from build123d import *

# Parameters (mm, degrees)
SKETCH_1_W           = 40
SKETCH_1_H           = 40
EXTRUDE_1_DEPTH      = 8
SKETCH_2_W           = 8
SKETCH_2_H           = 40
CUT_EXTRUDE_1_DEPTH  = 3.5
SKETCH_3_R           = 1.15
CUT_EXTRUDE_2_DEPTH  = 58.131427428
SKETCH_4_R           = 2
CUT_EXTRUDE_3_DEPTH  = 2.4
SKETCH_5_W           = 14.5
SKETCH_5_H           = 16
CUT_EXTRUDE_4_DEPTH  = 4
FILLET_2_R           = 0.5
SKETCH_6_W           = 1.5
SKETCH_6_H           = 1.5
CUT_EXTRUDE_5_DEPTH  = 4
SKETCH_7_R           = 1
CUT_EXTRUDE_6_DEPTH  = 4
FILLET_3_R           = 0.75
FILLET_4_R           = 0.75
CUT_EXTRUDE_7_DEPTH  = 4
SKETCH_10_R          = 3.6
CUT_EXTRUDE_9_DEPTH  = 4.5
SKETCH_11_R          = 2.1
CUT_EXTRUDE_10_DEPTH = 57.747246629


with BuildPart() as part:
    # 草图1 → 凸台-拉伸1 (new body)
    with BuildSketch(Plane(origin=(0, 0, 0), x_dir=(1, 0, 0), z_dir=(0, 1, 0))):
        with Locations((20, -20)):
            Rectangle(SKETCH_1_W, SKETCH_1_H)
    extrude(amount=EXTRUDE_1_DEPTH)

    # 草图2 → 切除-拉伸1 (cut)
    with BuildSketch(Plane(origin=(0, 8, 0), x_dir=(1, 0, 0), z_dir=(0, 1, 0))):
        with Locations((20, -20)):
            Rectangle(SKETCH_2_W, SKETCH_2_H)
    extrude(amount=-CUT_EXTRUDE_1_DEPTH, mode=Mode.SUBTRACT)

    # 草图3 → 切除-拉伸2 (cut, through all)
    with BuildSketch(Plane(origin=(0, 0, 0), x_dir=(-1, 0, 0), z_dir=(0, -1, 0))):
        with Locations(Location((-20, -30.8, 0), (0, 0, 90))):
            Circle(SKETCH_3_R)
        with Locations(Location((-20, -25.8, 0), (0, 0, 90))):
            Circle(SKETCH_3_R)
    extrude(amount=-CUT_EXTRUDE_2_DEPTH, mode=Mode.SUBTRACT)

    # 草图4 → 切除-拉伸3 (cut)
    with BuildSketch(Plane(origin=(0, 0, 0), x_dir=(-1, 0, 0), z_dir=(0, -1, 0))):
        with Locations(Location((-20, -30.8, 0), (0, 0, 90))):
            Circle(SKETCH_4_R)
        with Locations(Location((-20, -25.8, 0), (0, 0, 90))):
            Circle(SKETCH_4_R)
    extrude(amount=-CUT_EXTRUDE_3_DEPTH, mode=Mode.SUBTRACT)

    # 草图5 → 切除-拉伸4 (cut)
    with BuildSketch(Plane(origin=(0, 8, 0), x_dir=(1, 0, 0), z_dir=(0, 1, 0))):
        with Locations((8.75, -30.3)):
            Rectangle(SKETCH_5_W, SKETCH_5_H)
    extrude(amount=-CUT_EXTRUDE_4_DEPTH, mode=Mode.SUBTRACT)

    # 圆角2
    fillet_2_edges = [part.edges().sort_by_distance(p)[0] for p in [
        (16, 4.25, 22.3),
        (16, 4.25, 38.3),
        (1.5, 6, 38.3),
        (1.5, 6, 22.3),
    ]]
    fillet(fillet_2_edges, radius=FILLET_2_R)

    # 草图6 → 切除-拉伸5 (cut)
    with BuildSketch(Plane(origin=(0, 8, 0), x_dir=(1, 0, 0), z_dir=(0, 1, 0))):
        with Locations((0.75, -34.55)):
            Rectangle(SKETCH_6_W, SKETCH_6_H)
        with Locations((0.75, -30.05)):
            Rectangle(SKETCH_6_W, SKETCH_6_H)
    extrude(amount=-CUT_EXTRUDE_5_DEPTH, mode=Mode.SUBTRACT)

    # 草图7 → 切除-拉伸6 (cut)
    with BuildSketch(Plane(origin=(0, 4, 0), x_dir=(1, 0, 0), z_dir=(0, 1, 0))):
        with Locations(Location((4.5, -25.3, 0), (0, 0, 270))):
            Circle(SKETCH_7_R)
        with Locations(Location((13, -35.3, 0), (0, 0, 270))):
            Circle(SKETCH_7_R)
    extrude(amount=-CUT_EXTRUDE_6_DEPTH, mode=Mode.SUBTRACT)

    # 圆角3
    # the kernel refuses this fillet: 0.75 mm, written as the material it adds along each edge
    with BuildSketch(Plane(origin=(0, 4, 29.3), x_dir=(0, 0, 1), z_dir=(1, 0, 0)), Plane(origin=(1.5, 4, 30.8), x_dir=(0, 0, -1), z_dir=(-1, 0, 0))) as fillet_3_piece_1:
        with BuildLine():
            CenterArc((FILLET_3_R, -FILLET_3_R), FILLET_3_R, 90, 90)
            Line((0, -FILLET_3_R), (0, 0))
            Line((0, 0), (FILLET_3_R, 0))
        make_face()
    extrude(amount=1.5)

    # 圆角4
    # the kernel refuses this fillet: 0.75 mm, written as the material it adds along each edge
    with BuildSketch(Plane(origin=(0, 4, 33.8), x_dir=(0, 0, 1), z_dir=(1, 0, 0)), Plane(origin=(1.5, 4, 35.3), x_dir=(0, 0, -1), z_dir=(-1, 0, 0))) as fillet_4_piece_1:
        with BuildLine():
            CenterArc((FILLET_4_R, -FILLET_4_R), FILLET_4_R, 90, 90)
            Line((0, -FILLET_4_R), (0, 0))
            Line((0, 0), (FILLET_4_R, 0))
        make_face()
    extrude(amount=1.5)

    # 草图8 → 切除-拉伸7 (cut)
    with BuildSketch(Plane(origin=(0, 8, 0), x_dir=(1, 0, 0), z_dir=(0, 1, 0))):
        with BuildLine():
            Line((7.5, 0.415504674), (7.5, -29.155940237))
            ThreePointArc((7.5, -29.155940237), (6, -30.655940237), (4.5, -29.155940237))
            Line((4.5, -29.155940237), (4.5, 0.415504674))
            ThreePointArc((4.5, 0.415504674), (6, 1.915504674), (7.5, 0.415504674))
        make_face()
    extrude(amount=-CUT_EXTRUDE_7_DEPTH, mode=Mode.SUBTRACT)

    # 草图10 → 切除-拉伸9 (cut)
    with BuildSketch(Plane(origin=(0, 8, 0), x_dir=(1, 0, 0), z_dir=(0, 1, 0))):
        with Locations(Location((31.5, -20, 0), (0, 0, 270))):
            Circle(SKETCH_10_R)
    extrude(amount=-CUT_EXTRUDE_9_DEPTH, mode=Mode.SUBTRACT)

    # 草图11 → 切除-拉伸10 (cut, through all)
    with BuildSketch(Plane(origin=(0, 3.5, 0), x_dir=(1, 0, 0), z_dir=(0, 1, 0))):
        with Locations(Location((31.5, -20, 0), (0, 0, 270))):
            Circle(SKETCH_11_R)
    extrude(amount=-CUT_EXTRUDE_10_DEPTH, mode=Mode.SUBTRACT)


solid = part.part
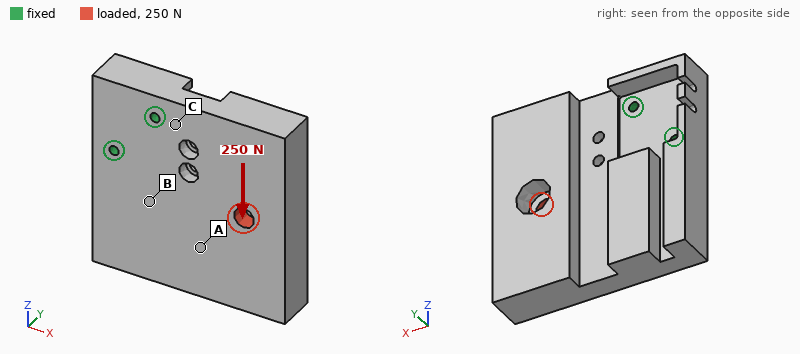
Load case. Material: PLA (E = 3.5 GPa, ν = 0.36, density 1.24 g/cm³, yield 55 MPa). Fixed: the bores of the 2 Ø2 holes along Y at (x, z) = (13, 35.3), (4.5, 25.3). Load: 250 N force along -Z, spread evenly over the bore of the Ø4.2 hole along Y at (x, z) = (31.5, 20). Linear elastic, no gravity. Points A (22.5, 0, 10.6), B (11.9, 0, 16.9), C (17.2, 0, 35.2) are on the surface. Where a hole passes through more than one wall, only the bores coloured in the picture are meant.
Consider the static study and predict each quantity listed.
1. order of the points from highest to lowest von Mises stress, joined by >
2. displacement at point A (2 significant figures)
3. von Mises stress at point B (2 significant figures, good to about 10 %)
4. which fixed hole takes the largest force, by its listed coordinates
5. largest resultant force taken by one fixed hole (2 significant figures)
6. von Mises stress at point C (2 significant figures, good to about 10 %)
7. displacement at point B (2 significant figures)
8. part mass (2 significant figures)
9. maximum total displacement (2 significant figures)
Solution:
C > B > A
0.14 mm
3.7 MPa
(13, 35.3)
490 N
7.7 MPa
0.067 mm
13 g
0.25 mm
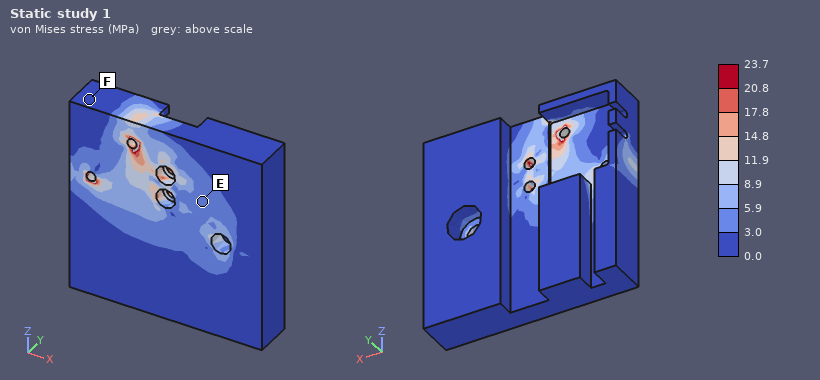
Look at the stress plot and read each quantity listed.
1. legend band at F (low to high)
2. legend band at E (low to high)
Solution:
0.0 to 3.0 MPa
3.0 to 5.9 MPa
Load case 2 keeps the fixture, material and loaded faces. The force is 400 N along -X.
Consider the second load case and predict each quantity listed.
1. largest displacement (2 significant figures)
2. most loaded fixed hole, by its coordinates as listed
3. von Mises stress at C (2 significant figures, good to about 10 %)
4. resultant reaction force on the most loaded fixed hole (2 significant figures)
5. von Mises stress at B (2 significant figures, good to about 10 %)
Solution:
0.22 mm
(4.5, 25.3)
4.5 MPa
460 N
6.3 MPa
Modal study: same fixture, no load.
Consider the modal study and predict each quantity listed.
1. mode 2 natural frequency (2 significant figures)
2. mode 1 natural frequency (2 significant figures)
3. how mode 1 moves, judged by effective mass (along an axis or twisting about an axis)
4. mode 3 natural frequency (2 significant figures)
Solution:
1500 Hz
620 Hz
along Y
2000 Hz
